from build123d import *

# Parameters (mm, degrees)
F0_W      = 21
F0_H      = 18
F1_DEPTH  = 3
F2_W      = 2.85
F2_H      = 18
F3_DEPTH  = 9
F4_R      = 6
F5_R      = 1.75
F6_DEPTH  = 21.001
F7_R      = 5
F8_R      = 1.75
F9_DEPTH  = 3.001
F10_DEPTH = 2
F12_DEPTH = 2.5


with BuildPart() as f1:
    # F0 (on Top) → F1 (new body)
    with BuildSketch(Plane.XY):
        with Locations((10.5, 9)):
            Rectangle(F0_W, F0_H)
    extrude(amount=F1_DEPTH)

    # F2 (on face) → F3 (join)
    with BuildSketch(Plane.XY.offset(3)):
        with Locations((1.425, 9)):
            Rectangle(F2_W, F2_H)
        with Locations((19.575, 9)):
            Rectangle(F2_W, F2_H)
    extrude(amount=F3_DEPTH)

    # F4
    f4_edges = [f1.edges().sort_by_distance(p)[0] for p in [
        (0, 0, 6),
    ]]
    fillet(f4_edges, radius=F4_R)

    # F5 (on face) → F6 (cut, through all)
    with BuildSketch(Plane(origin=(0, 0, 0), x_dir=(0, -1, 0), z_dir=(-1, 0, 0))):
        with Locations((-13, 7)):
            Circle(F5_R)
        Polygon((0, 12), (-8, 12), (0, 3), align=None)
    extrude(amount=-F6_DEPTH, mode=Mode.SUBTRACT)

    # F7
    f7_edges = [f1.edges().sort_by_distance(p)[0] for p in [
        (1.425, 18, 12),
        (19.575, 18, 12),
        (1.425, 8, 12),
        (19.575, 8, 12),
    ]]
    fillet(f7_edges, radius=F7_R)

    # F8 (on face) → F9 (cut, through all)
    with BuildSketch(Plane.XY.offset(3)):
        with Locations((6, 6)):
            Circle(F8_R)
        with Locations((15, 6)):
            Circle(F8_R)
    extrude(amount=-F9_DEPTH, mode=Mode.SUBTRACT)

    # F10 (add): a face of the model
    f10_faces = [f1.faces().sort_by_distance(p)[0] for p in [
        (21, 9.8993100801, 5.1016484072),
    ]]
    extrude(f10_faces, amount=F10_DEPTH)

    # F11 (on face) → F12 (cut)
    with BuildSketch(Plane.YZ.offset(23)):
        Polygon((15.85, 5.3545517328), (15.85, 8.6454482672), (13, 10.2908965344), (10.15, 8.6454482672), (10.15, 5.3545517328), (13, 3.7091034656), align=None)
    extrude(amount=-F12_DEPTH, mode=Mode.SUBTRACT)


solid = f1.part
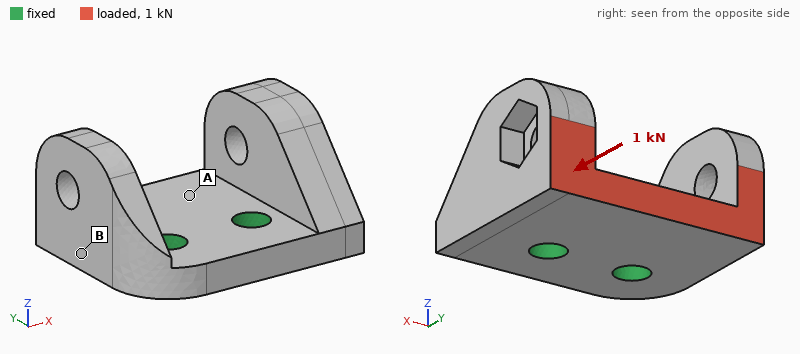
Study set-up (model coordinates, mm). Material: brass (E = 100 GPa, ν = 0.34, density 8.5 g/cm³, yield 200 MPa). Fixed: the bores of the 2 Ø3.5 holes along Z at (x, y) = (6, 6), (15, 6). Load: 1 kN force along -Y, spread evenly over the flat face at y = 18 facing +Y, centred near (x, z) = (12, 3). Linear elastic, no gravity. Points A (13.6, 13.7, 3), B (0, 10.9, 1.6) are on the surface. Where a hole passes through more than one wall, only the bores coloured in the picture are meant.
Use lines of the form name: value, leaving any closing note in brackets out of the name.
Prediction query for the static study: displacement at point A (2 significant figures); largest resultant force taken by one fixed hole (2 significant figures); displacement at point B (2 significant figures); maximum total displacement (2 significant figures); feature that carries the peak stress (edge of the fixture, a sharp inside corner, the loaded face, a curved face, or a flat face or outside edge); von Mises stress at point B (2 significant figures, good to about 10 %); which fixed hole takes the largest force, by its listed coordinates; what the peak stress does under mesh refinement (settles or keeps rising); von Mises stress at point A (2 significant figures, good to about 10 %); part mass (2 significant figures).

displacement at point A: 2.6 µm
largest resultant force taken by one fixed hole: 630 N
displacement at point B: 1.5 µm
maximum total displacement: 7.7 µm
feature that carries the peak stress: edge of the fixture
von Mises stress at point B: 6.2 MPa
which fixed hole takes the largest force, by its listed coordinates: (15, 6)
what the peak stress does under mesh refinement: keeps rising
von Mises stress at point A: 15 MPa
part mass: 17 g
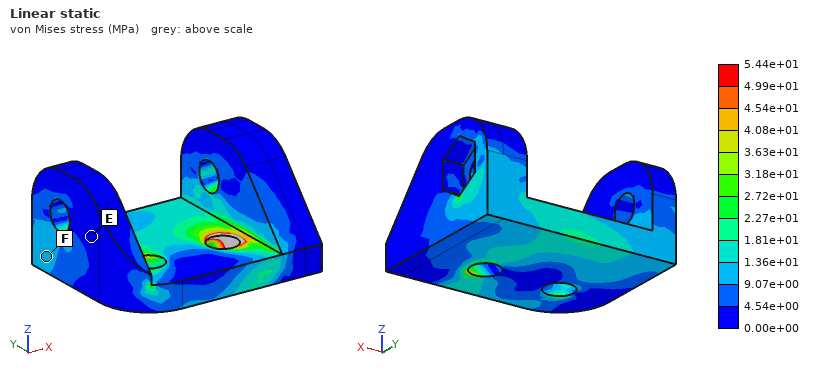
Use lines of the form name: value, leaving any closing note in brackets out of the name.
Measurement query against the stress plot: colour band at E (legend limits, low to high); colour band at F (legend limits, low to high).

colour band at E: 0.00e+00 to 4.54e+00 MPa
colour band at F: 9.07e+00 to 1.36e+01 MPa
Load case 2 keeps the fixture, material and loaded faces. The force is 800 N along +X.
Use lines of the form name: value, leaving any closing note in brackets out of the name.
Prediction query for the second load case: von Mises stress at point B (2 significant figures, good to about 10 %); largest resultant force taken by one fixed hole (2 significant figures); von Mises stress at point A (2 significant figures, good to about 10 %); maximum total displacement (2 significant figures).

von Mises stress at point B: 20 MPa
largest resultant force taken by one fixed hole: 840 N
von Mises stress at point A: 41 MPa
maximum total displacement: 18 µm
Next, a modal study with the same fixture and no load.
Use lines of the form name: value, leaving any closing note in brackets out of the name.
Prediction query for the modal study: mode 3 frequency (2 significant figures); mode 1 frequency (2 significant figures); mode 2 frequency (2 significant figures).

mode 3 frequency: 11 kHz
mode 1 frequency: 8200 Hz
mode 2 frequency: 9700 Hz
